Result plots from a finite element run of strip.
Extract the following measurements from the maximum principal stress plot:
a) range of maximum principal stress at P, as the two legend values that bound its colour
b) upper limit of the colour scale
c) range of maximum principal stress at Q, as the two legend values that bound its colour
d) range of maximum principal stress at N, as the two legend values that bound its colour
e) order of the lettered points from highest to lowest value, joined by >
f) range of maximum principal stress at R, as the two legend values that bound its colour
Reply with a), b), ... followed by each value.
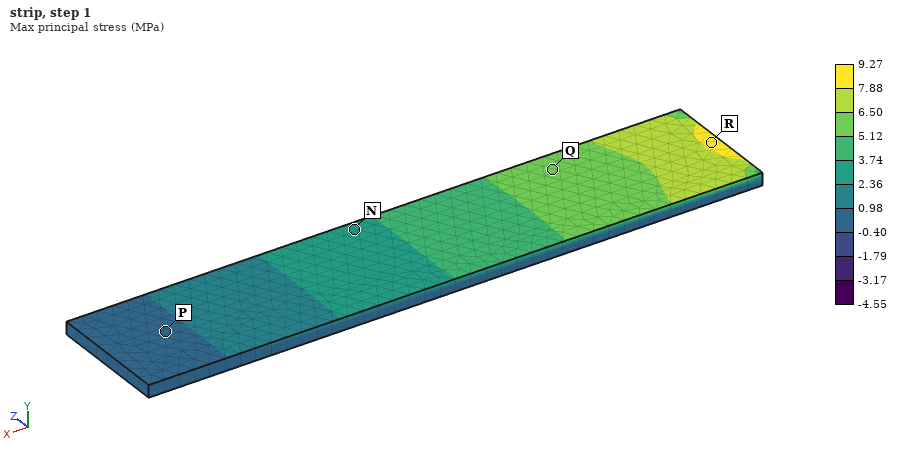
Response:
a) -0.40 to 0.98 MPa
b) 9.27 MPa
c) 5.12 to 6.50 MPa
d) 2.36 to 3.74 MPa
e) R > Q > N > P
f) 7.88 to 9.27 MPa
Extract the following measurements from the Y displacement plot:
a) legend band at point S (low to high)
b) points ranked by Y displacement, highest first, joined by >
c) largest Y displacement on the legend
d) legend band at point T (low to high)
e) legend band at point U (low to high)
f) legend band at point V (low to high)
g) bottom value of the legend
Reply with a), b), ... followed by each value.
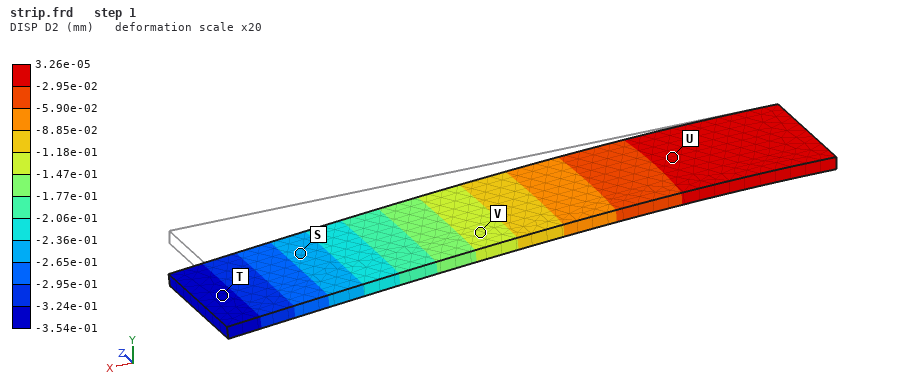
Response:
a) -2.65e-01 to -2.36e-01 mm
b) U > V > S > T
c) 3.26e-05 mm
d) -3.54e-01 to -3.24e-01 mm
e) -2.95e-02 to 3.26e-05 mm
f) -1.47e-01 to -1.18e-01 mm
g) -3.54e-01 mm
